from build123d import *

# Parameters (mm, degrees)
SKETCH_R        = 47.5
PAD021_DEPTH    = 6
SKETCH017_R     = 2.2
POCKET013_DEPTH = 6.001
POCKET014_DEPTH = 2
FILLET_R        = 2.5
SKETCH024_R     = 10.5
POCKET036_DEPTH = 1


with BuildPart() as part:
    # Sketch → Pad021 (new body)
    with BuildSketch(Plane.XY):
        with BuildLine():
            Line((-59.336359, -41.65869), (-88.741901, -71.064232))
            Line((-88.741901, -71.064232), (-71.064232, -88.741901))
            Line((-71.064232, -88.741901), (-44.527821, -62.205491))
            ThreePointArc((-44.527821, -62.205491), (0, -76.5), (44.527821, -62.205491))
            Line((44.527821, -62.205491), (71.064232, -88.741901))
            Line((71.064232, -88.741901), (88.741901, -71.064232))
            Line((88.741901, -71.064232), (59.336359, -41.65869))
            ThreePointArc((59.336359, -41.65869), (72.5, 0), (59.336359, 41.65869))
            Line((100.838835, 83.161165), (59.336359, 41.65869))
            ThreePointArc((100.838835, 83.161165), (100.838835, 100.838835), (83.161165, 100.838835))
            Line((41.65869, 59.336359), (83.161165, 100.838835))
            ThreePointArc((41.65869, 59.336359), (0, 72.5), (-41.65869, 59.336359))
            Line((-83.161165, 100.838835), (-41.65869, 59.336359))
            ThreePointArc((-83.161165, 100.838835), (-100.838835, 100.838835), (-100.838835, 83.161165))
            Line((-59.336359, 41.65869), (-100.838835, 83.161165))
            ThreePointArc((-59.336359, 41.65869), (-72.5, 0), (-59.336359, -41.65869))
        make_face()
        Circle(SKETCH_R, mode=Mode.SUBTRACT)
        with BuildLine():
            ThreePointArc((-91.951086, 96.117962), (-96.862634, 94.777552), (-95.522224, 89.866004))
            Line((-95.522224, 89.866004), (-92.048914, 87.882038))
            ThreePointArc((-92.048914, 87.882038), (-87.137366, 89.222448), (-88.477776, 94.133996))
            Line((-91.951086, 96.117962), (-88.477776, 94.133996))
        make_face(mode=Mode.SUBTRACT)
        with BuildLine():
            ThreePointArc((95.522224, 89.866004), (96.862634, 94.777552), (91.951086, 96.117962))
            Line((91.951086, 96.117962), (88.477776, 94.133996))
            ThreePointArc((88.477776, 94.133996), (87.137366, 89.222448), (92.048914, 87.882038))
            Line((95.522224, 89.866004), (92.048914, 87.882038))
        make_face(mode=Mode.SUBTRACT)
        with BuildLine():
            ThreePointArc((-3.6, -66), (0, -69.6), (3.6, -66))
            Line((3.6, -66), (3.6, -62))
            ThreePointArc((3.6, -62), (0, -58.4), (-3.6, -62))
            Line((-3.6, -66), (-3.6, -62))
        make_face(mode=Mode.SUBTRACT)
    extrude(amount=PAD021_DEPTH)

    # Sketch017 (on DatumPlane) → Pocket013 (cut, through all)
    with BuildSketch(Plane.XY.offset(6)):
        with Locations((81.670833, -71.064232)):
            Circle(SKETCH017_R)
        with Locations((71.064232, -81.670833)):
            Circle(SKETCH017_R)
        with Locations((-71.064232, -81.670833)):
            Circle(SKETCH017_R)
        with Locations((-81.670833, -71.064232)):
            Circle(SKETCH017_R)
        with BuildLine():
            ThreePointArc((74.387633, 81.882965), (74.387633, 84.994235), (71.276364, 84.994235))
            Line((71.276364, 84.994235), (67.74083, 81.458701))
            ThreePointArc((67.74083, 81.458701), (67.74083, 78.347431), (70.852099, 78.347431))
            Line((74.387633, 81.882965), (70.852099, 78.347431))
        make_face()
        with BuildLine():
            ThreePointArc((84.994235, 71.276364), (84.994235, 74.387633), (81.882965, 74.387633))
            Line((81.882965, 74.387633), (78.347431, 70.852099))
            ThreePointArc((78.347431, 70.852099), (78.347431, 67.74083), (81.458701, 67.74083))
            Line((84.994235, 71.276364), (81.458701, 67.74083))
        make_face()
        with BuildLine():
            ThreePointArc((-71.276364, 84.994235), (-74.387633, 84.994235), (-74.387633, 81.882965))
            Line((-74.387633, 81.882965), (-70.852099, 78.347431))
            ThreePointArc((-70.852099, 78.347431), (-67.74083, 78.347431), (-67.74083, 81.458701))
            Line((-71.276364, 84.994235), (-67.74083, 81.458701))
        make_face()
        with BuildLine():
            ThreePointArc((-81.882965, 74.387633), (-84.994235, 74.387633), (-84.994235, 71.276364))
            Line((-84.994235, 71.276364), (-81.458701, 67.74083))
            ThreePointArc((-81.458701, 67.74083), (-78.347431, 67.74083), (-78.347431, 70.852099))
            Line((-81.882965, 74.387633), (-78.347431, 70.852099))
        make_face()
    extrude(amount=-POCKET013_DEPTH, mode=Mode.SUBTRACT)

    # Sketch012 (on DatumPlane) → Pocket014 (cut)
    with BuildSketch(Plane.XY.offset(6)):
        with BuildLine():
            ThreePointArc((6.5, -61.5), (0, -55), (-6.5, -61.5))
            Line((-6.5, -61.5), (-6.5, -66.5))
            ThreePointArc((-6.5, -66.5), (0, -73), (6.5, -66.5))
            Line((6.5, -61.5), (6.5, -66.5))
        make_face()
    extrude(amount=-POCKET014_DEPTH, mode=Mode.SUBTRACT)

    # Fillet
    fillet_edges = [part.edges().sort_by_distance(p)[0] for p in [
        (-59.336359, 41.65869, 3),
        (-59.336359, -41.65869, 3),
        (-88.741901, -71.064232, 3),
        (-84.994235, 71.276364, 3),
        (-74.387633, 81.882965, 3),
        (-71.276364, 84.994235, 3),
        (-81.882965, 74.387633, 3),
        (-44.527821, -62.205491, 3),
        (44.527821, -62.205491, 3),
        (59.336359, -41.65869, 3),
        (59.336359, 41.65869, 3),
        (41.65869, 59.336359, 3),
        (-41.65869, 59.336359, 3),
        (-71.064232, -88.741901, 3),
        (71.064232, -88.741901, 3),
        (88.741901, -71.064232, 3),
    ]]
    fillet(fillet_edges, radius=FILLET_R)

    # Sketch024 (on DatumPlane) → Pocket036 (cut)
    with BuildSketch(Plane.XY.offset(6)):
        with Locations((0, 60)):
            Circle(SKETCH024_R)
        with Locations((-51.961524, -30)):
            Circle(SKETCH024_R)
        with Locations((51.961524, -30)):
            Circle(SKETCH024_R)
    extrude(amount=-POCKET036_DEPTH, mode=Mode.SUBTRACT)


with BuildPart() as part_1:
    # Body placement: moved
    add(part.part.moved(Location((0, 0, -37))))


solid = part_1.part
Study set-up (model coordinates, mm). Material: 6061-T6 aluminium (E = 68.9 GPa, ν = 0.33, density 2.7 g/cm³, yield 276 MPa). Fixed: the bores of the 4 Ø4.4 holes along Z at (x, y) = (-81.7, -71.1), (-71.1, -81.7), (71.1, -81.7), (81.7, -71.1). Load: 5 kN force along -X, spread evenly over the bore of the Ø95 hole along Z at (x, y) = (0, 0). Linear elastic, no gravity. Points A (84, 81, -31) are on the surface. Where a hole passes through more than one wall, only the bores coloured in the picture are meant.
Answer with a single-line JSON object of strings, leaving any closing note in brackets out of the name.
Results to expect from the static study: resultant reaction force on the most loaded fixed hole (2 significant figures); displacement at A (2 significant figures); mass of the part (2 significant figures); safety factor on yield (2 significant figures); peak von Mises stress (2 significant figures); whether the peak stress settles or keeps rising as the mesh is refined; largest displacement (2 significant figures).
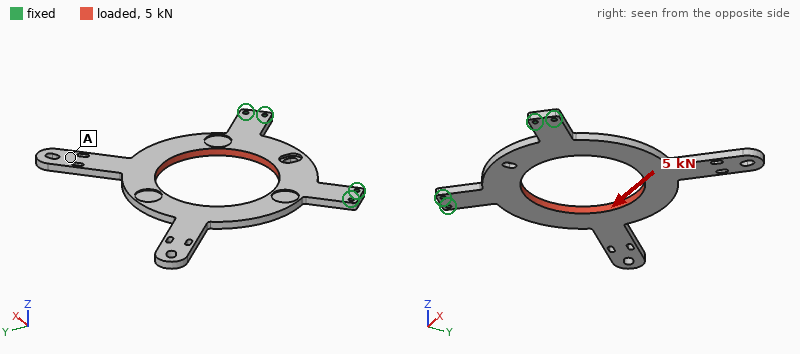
{"resultant reaction force on the most loaded fixed hole": "2.7 kN", "displacement at A": "0.32 mm", "mass of the part": "240 g", "safety factor on yield": "1.4", "peak von Mises stress": "200 MPa", "whether the peak stress settles or keeps rising as the mesh is refined": "settles", "largest displacement": "0.35 mm"}
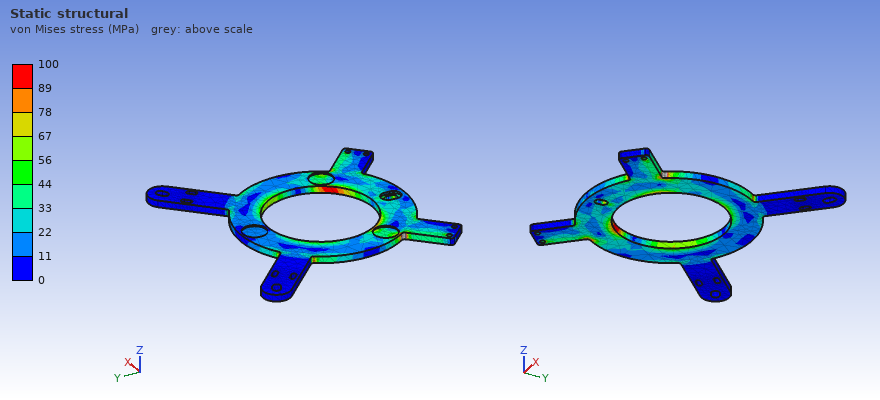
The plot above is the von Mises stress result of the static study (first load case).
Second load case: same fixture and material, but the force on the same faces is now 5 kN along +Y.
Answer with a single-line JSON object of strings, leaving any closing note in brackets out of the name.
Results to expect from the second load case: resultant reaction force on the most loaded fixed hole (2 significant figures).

{"resultant reaction force on the most loaded fixed hole": "2.6 kN"}
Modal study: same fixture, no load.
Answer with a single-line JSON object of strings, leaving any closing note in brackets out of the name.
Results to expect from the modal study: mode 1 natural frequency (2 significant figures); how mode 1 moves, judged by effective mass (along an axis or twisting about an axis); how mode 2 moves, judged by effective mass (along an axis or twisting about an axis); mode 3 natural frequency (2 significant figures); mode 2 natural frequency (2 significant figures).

{"mode 1 natural frequency": "120 Hz", "how mode 1 moves, judged by effective mass": "along Z", "how mode 2 moves, judged by effective mass": "twisting about Y", "mode 3 natural frequency": "670 Hz", "mode 2 natural frequency": "260 Hz"}
